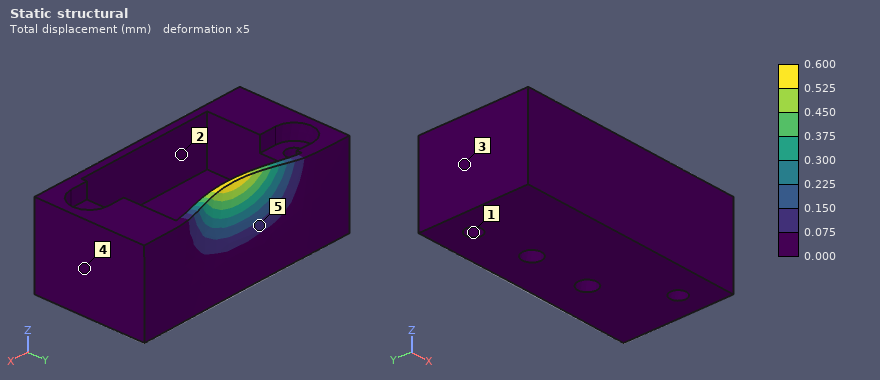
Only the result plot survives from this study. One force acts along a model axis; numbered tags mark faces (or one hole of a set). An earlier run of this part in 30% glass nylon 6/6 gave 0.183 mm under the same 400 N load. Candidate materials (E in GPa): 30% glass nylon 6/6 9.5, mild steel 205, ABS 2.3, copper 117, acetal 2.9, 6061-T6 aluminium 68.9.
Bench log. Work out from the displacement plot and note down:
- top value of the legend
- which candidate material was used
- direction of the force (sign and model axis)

0.600 mm
acetal
-Y
